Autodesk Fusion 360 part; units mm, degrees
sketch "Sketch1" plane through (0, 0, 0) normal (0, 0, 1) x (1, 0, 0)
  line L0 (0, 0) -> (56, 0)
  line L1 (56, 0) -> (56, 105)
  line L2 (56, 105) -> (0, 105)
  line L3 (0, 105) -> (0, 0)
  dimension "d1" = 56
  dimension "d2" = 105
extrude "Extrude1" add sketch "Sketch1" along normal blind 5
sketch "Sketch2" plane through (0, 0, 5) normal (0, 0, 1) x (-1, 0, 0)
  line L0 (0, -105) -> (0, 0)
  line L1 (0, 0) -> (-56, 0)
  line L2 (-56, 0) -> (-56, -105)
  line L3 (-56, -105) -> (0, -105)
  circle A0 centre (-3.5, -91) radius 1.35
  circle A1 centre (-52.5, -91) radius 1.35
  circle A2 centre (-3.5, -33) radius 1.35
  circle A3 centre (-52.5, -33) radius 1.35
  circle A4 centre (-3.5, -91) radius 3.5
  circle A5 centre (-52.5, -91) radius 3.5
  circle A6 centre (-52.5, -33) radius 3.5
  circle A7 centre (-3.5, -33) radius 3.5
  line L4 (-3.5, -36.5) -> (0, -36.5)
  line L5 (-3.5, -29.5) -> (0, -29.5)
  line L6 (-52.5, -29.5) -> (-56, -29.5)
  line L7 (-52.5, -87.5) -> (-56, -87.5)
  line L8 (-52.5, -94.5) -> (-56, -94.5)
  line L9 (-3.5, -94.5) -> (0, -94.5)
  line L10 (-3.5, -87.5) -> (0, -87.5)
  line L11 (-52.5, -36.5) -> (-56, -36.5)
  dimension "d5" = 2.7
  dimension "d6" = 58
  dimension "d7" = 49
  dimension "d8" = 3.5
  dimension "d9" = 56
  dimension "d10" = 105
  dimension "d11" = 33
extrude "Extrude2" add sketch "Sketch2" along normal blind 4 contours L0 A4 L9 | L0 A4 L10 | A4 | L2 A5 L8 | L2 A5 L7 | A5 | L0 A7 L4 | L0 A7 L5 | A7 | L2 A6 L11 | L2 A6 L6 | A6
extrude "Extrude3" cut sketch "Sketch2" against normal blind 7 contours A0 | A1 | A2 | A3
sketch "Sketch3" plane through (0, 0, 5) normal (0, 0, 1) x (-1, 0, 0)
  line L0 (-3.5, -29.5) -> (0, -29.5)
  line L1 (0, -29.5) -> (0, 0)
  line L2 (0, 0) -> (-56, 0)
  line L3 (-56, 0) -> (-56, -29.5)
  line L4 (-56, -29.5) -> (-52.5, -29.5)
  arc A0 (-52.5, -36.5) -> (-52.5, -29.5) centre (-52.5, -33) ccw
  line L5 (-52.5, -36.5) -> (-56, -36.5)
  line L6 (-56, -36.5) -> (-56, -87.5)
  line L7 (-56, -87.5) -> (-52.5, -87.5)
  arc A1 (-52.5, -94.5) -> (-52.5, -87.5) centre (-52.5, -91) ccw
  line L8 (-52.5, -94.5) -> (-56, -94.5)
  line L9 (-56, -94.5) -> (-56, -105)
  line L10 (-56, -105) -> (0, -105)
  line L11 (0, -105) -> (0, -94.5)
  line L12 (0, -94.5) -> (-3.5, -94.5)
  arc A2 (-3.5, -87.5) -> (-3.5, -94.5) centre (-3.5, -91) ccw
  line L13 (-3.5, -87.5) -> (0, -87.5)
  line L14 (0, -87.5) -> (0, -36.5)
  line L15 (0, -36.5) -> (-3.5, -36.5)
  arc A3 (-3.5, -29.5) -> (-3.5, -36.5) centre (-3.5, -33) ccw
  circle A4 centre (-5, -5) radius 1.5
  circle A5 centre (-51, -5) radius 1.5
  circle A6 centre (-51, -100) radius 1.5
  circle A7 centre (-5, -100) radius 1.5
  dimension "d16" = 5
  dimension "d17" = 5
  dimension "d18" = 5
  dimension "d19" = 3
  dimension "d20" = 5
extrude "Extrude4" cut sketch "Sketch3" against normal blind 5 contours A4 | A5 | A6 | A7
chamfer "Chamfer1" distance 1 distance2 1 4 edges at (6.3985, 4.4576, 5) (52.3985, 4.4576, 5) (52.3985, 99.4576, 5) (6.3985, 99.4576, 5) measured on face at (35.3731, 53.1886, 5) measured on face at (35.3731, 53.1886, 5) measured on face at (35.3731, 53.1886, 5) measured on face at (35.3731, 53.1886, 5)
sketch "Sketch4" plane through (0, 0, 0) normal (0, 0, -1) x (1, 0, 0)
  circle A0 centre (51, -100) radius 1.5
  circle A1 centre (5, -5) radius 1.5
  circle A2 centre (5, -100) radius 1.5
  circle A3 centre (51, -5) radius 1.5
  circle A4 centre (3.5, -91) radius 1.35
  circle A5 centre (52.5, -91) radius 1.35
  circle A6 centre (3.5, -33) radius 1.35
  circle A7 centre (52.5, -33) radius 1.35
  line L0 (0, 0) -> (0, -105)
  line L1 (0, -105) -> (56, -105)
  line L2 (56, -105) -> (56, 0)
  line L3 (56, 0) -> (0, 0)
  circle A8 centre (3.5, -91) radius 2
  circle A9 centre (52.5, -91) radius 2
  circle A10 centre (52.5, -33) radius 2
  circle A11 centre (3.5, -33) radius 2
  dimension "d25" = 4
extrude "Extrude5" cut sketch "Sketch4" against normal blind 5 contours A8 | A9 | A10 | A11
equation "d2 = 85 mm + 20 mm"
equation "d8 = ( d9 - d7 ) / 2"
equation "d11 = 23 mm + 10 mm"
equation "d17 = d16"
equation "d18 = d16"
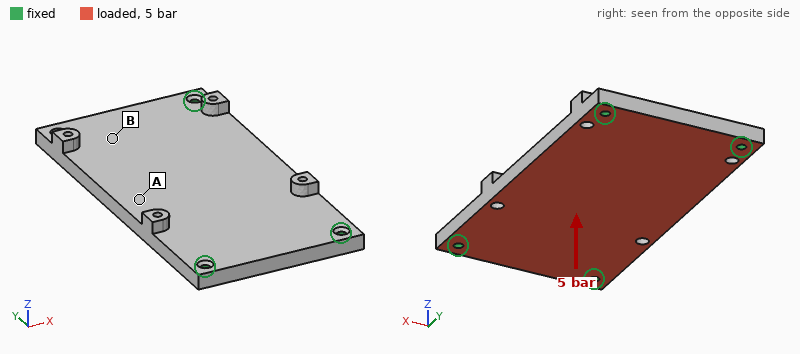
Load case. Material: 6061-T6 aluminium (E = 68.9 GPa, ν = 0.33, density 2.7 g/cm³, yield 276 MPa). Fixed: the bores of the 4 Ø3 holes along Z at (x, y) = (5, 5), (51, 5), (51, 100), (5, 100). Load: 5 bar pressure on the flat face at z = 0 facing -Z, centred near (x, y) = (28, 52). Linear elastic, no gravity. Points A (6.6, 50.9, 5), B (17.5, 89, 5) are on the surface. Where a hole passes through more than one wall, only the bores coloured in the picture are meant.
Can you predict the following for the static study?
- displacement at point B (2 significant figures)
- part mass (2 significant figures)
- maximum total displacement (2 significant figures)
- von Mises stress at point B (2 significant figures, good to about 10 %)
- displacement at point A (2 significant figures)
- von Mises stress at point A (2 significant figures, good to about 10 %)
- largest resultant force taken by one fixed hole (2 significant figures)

0.075 mm
80 g
0.24 mm
22 MPa
0.23 mm
59 MPa
740 N
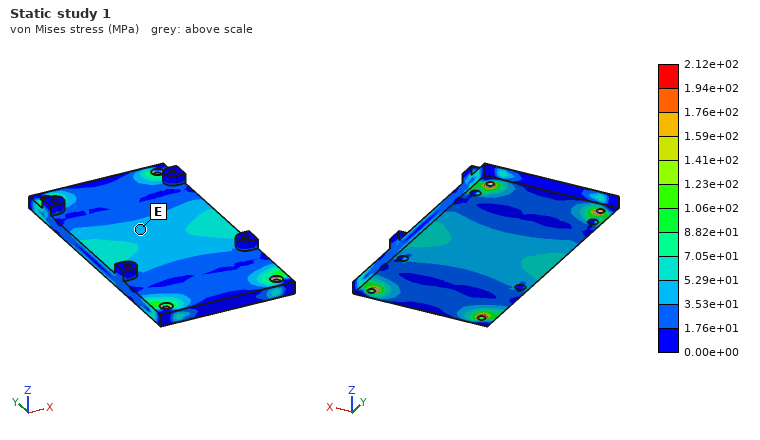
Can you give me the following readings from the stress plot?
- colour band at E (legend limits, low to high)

3.53e+01 to 5.29e+01 MPa
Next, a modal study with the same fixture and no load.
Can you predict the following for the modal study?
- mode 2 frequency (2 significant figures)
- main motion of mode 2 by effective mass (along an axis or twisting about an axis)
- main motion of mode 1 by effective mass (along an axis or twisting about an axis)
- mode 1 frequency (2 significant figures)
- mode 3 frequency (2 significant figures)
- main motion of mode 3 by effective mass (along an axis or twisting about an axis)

3900 Hz
twisting about Y
along Z
2300 Hz
6200 Hz
twisting about X
